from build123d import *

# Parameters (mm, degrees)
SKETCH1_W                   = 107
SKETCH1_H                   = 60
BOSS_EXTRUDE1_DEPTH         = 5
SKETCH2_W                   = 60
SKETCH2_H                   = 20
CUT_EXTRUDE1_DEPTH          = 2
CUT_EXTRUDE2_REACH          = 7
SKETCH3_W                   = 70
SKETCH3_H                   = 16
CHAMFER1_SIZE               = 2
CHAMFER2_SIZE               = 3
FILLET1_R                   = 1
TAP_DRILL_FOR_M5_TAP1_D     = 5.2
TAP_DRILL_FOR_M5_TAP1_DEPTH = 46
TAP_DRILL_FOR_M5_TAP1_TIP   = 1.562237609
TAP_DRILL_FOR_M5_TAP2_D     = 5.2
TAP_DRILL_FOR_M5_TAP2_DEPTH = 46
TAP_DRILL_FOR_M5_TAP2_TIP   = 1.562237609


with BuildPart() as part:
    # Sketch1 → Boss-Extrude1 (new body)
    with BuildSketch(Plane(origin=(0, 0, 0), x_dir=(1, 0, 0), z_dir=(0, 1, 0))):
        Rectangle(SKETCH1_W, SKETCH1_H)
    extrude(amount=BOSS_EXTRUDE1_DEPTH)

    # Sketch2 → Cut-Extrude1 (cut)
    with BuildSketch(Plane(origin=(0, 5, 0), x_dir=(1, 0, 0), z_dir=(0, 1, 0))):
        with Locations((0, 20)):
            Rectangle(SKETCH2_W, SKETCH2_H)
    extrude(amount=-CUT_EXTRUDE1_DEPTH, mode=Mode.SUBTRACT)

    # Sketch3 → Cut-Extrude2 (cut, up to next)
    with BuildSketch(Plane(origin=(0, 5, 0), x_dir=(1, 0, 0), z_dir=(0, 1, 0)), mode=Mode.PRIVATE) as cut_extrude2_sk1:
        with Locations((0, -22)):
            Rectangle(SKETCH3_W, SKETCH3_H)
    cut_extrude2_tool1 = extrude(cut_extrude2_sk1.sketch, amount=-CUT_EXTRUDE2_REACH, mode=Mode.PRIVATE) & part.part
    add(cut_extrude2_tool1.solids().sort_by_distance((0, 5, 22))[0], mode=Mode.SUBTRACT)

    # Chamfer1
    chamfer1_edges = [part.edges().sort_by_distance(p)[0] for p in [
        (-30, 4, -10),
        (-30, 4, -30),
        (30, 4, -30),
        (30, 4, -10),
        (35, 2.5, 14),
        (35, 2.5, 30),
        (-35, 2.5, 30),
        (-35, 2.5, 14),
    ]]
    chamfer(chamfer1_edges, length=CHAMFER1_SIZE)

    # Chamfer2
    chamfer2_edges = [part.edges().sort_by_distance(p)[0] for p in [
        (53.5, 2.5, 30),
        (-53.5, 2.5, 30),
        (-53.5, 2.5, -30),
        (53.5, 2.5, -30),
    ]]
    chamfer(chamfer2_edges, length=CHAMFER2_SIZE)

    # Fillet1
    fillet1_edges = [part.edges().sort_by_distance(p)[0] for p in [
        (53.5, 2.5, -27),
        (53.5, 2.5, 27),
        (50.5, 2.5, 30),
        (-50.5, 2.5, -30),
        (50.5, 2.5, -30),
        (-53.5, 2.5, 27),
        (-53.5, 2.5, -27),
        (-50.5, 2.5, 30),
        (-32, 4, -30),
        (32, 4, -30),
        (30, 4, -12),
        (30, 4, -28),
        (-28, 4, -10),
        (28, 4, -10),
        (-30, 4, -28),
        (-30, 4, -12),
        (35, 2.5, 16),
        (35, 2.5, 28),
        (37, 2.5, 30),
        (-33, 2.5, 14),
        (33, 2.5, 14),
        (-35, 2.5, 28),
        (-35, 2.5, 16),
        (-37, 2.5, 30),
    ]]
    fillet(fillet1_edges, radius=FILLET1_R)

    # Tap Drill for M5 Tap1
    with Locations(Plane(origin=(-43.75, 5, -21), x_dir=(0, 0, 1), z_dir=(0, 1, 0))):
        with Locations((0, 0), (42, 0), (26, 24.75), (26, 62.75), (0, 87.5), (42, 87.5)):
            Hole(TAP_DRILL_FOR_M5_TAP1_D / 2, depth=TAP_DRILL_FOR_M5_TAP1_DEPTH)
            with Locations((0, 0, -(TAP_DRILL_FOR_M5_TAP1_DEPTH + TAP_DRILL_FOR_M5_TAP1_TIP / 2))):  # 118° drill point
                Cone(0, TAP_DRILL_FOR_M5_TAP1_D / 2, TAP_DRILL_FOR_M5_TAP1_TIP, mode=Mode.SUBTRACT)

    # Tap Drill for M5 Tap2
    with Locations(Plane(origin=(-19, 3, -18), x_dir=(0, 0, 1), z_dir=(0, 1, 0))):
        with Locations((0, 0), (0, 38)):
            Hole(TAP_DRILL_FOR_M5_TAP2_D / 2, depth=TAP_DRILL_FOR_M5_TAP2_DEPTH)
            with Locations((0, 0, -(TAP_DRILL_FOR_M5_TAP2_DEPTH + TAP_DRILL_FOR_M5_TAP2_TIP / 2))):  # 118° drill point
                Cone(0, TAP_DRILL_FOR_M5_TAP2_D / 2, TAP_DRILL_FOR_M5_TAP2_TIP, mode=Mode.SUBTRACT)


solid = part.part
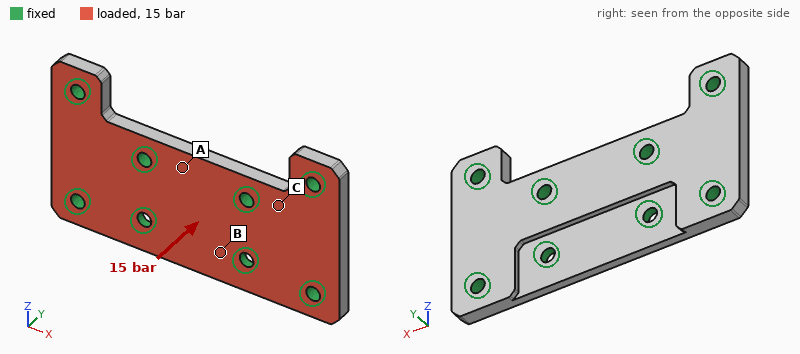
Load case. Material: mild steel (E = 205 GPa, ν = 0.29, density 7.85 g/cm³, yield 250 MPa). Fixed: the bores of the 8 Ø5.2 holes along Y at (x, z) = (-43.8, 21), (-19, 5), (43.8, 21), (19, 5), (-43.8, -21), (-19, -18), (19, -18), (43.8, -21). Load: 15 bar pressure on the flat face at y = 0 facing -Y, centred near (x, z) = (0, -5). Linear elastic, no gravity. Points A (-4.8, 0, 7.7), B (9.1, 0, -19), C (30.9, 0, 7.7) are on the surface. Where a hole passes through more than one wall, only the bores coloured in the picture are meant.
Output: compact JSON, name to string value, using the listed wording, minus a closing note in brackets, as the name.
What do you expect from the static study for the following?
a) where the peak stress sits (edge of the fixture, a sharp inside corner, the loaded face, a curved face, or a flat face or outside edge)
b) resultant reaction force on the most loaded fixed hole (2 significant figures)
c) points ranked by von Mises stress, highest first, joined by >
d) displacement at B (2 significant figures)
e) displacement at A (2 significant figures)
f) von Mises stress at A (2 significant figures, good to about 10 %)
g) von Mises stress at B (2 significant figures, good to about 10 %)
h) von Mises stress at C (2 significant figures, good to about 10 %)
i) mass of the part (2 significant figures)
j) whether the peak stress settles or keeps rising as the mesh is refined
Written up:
{"where the peak stress sits": "edge of the fixture", "resultant reaction force on the most loaded fixed hole": "1.1 kN", "points ranked by von Mises stress, highest first, joined by >": "B > A > C", "displacement at B": "7.8 µm", "displacement at A": "3.5 µm", "von Mises stress at A": "16 MPa", "von Mises stress at B": "33 MPa", "von Mises stress at C": "8.9 MPa", "mass of the part": "180 g", "whether the peak stress settles or keeps rising as the mesh is refined": "keeps rising"}
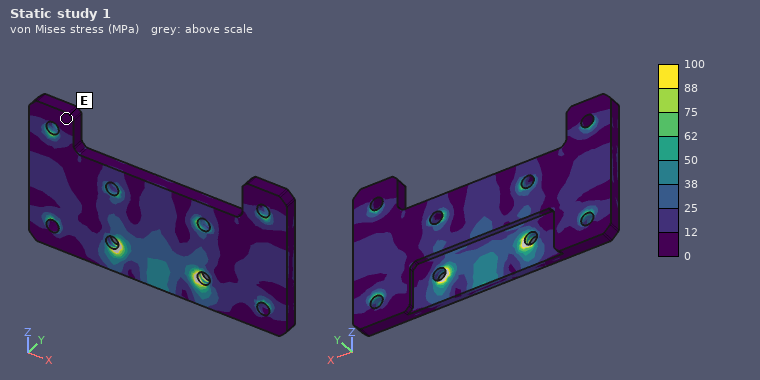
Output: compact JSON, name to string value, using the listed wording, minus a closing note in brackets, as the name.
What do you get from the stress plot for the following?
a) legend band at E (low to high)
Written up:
{"legend band at E": "0 to 12 MPa"}
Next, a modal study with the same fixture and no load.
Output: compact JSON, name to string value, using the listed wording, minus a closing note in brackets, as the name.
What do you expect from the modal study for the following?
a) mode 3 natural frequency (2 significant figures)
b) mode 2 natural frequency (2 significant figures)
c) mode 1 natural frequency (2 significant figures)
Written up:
{"mode 3 natural frequency": "15 kHz", "mode 2 natural frequency": "15 kHz", "mode 1 natural frequency": "11 kHz"}
